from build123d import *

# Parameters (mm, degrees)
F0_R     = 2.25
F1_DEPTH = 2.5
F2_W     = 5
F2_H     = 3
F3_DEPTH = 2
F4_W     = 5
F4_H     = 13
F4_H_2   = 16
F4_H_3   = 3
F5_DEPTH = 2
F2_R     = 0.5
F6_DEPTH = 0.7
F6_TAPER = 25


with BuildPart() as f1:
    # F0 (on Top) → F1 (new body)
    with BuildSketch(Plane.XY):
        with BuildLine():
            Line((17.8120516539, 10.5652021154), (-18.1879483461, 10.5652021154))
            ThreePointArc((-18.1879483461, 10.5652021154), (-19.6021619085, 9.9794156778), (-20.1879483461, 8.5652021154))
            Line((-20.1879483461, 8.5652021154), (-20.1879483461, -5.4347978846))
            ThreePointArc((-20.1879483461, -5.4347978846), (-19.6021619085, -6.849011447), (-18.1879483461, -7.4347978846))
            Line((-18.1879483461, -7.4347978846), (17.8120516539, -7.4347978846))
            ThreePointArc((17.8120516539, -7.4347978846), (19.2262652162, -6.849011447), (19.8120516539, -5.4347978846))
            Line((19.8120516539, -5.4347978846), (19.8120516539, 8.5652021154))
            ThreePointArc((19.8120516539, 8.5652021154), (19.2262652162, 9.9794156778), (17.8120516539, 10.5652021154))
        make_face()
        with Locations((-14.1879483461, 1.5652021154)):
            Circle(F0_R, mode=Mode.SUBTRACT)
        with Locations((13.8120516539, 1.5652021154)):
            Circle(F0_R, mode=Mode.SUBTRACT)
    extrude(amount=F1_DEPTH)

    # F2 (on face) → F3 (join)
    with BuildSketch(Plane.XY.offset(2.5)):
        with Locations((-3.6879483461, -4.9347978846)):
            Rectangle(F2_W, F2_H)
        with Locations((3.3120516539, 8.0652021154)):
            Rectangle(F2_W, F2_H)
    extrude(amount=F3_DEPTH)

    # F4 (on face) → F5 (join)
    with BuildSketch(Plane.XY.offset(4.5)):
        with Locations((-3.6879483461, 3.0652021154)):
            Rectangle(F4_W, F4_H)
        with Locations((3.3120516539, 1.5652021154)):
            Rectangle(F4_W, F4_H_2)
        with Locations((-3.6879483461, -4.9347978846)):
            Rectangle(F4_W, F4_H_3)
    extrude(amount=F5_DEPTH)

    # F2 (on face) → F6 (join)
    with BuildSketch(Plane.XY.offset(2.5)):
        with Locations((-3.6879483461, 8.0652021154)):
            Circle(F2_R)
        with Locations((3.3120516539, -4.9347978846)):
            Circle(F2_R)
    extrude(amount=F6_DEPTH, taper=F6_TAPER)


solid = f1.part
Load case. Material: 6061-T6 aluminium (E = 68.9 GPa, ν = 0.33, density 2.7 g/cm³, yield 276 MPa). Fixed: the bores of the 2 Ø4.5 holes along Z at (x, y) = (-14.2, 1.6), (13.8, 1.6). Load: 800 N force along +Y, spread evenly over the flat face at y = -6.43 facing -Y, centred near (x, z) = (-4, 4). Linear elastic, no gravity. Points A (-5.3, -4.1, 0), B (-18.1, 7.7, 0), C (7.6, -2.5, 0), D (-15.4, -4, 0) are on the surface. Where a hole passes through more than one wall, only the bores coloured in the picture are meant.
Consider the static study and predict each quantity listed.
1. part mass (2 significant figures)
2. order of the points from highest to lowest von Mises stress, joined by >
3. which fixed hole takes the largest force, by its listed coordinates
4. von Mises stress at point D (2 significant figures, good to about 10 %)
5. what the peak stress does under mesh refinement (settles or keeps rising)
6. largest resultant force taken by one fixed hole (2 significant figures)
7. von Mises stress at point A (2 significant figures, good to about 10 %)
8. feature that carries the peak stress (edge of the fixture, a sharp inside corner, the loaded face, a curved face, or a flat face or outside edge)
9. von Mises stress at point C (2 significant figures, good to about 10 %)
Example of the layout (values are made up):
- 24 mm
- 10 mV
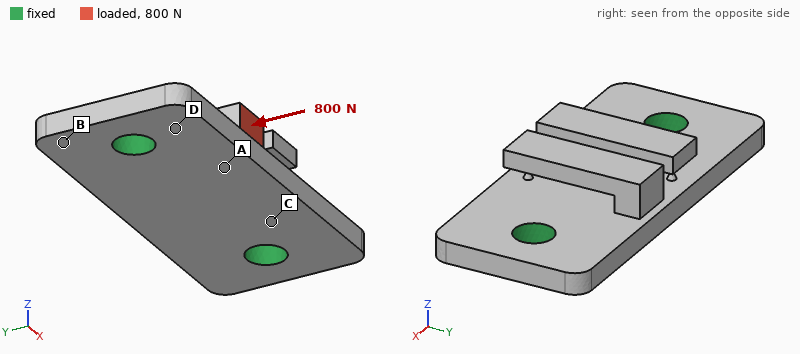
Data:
- 5.6 g
- A > D > C > B
- (-14.2, 1.6)
- 61 MPa
- keeps rising
- 520 N
- 110 MPa
- a sharp inside corner
- 43 MPa
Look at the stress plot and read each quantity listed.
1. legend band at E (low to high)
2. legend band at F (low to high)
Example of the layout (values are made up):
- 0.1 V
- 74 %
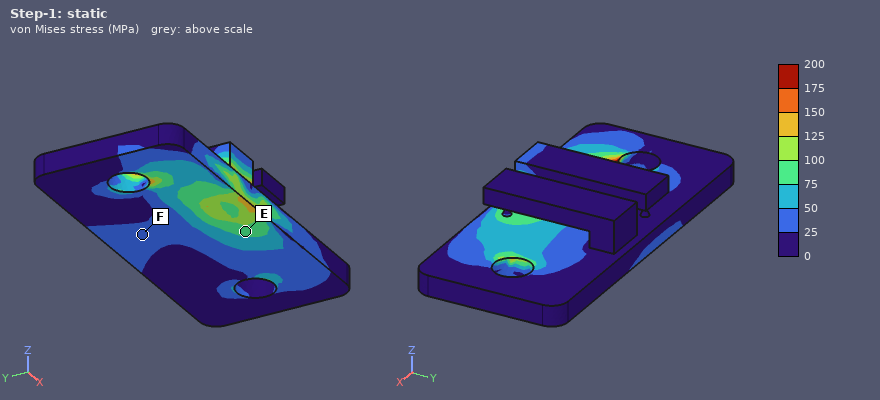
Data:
- 75 to 100 MPa
- 25 to 50 MPa
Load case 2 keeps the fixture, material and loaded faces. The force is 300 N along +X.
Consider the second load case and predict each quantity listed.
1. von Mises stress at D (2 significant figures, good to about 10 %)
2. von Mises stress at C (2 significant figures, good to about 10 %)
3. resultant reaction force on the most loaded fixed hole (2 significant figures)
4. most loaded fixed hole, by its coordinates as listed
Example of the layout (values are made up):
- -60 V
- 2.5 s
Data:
- 7.9 MPa
- 12 MPa
- 200 N
- (-14.2, 1.6)
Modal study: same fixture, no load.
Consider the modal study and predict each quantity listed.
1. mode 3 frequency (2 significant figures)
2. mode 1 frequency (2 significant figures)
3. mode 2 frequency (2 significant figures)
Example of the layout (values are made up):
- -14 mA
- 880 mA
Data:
- 11 kHz
- 6800 Hz
- 6900 Hz
